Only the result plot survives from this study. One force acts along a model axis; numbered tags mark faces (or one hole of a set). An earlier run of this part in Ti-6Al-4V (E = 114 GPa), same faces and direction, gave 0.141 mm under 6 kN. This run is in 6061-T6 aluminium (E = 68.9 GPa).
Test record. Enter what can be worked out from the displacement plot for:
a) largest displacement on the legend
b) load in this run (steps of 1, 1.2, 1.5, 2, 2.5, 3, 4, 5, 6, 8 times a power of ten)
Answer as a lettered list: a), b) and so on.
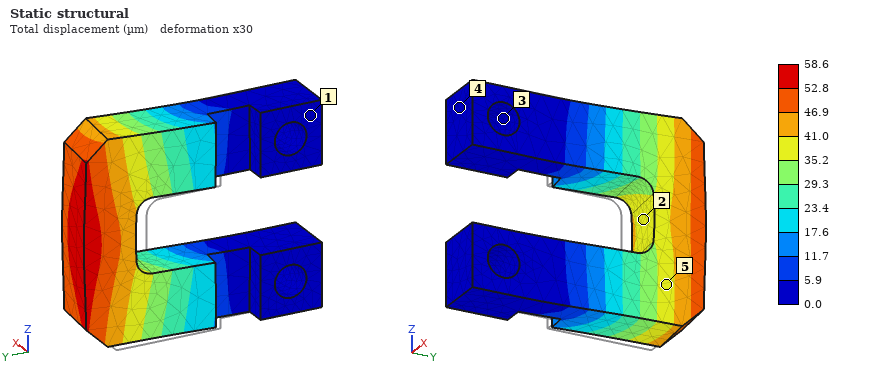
a) 58.6 µm
b) 1.5 kN
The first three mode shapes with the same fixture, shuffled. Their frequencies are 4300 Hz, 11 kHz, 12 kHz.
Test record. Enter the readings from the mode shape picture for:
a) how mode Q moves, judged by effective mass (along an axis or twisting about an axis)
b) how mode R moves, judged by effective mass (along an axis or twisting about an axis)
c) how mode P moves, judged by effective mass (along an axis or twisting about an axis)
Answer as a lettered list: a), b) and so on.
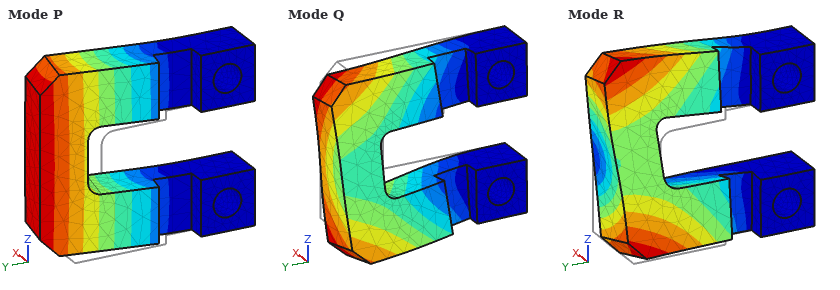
a) along Z
b) along Z
c) along X
